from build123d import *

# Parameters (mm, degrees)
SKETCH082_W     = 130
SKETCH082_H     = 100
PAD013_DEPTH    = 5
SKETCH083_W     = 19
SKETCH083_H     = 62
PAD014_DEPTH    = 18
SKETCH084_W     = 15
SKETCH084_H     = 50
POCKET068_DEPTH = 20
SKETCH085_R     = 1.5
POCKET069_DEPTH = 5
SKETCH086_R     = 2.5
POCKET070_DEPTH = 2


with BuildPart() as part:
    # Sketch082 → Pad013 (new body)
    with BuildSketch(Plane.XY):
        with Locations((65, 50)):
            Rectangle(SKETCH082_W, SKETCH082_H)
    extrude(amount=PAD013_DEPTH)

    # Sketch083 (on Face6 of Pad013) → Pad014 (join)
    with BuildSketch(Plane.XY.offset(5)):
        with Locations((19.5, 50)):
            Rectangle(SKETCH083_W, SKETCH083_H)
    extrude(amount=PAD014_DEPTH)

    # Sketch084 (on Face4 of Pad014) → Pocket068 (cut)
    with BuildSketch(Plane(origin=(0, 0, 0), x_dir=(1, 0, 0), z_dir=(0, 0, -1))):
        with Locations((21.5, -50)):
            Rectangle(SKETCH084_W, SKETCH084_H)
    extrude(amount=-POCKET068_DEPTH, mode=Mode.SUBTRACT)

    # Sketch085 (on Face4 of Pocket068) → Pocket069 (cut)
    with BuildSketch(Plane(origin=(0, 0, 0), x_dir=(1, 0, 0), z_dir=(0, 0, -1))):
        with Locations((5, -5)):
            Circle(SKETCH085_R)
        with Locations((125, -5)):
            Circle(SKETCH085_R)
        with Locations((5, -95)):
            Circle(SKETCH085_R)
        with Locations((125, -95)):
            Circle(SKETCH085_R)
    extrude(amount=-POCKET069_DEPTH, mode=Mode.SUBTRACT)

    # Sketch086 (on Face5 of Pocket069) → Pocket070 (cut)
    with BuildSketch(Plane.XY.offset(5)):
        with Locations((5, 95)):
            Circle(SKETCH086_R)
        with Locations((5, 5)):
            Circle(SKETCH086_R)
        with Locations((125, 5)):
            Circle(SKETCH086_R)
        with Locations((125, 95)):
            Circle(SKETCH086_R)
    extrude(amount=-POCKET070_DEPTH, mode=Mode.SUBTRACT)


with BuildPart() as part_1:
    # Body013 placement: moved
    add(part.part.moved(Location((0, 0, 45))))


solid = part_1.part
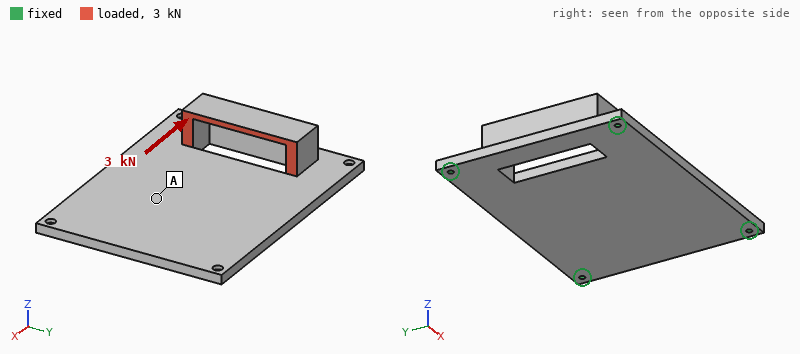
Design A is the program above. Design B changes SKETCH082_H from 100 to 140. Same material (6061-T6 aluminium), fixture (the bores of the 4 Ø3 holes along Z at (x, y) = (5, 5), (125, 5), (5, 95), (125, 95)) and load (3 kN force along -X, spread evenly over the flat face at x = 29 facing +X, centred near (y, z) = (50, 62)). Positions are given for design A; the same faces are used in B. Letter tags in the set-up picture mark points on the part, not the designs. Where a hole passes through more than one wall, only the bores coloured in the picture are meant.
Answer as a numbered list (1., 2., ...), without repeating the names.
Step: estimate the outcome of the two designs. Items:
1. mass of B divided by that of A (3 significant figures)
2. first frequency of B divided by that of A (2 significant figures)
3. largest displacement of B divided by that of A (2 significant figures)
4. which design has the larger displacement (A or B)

1. 1.37
2. 1.0
3. 0.84
4. A
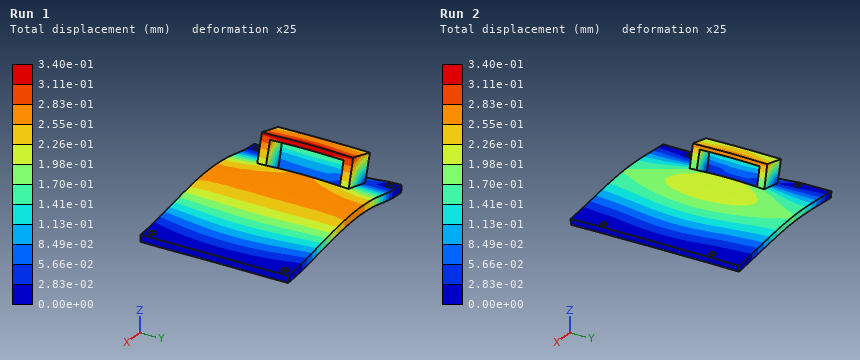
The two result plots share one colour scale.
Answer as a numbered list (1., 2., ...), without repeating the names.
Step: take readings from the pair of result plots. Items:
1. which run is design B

1. Run 2
